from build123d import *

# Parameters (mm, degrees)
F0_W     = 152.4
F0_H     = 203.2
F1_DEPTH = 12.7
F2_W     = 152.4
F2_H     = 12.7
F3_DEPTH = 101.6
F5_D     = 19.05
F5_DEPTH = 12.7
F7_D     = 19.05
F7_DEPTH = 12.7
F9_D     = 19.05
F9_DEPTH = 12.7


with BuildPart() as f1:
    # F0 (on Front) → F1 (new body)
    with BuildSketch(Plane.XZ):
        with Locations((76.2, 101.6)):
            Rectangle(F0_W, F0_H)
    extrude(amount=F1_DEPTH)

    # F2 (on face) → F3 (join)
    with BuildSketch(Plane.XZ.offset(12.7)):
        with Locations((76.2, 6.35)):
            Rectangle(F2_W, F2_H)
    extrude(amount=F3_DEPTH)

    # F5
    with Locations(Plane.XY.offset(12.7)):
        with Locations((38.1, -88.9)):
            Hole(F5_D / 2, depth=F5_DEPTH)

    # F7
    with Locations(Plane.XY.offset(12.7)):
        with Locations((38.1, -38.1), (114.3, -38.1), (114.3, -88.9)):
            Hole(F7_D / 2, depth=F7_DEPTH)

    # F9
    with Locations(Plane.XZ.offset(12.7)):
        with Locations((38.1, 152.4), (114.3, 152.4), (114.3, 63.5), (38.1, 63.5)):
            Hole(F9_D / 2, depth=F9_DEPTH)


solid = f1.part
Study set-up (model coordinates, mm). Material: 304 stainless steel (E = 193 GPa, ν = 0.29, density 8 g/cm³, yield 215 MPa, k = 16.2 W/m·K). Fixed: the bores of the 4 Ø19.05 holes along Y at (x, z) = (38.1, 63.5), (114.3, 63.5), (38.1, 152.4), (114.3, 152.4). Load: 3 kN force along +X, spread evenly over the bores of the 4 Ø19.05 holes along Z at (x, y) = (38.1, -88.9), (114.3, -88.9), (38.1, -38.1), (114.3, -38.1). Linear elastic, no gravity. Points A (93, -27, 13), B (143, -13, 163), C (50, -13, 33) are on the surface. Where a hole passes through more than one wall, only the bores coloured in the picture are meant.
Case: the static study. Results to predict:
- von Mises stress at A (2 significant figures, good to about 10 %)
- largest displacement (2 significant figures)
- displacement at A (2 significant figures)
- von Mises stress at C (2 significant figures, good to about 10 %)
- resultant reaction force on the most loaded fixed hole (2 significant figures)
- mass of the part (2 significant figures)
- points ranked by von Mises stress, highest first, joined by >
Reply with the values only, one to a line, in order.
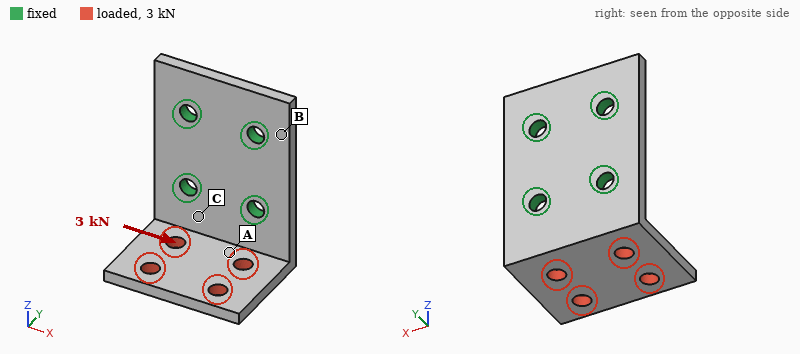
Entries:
12 MPa
61 µm
13 µm
18 MPa
2.8 kN
4.5 kg
C > A > B
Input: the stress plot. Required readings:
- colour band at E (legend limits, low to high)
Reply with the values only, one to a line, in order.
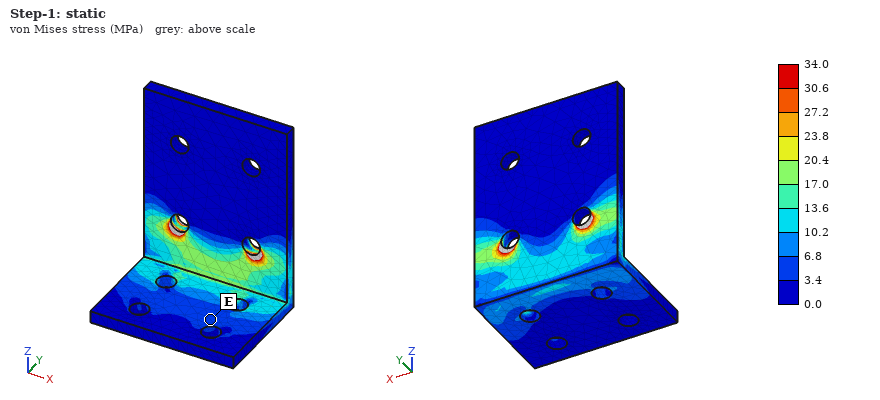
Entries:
3.4 to 6.8 MPa
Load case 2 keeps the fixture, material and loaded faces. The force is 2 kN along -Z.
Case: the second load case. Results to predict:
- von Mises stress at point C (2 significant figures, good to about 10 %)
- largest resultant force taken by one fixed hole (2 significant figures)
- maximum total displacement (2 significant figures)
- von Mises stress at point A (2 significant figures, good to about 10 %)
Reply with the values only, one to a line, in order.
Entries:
27 MPa
920 N
0.19 mm
20 MPa
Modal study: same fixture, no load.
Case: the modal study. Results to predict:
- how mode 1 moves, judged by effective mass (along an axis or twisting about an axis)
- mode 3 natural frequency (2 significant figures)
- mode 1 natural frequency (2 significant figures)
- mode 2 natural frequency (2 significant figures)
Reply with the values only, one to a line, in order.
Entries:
along Z
1500 Hz
500 Hz
970 Hz
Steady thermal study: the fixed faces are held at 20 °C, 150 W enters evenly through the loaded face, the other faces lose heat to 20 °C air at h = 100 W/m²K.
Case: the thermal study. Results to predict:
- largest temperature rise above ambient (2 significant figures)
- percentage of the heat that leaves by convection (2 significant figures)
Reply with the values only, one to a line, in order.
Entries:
68 K
96 %
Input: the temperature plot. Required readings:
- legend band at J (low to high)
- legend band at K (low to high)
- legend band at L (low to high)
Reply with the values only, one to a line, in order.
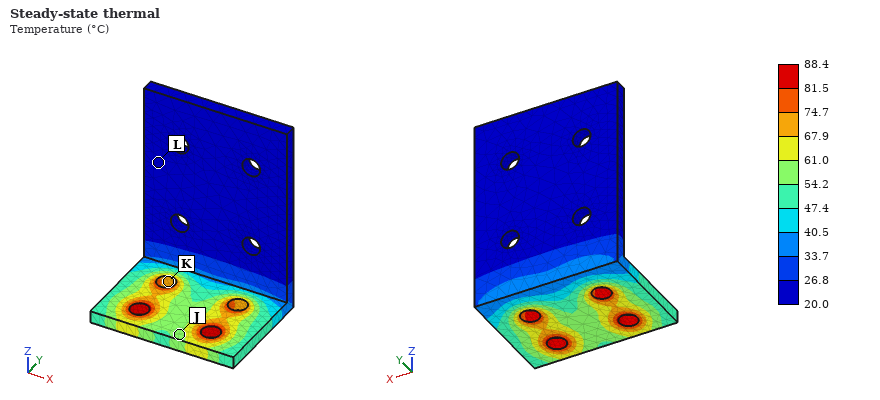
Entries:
54.2 to 61.0 °C
67.9 to 74.7 °C
20.0 to 26.8 °C
